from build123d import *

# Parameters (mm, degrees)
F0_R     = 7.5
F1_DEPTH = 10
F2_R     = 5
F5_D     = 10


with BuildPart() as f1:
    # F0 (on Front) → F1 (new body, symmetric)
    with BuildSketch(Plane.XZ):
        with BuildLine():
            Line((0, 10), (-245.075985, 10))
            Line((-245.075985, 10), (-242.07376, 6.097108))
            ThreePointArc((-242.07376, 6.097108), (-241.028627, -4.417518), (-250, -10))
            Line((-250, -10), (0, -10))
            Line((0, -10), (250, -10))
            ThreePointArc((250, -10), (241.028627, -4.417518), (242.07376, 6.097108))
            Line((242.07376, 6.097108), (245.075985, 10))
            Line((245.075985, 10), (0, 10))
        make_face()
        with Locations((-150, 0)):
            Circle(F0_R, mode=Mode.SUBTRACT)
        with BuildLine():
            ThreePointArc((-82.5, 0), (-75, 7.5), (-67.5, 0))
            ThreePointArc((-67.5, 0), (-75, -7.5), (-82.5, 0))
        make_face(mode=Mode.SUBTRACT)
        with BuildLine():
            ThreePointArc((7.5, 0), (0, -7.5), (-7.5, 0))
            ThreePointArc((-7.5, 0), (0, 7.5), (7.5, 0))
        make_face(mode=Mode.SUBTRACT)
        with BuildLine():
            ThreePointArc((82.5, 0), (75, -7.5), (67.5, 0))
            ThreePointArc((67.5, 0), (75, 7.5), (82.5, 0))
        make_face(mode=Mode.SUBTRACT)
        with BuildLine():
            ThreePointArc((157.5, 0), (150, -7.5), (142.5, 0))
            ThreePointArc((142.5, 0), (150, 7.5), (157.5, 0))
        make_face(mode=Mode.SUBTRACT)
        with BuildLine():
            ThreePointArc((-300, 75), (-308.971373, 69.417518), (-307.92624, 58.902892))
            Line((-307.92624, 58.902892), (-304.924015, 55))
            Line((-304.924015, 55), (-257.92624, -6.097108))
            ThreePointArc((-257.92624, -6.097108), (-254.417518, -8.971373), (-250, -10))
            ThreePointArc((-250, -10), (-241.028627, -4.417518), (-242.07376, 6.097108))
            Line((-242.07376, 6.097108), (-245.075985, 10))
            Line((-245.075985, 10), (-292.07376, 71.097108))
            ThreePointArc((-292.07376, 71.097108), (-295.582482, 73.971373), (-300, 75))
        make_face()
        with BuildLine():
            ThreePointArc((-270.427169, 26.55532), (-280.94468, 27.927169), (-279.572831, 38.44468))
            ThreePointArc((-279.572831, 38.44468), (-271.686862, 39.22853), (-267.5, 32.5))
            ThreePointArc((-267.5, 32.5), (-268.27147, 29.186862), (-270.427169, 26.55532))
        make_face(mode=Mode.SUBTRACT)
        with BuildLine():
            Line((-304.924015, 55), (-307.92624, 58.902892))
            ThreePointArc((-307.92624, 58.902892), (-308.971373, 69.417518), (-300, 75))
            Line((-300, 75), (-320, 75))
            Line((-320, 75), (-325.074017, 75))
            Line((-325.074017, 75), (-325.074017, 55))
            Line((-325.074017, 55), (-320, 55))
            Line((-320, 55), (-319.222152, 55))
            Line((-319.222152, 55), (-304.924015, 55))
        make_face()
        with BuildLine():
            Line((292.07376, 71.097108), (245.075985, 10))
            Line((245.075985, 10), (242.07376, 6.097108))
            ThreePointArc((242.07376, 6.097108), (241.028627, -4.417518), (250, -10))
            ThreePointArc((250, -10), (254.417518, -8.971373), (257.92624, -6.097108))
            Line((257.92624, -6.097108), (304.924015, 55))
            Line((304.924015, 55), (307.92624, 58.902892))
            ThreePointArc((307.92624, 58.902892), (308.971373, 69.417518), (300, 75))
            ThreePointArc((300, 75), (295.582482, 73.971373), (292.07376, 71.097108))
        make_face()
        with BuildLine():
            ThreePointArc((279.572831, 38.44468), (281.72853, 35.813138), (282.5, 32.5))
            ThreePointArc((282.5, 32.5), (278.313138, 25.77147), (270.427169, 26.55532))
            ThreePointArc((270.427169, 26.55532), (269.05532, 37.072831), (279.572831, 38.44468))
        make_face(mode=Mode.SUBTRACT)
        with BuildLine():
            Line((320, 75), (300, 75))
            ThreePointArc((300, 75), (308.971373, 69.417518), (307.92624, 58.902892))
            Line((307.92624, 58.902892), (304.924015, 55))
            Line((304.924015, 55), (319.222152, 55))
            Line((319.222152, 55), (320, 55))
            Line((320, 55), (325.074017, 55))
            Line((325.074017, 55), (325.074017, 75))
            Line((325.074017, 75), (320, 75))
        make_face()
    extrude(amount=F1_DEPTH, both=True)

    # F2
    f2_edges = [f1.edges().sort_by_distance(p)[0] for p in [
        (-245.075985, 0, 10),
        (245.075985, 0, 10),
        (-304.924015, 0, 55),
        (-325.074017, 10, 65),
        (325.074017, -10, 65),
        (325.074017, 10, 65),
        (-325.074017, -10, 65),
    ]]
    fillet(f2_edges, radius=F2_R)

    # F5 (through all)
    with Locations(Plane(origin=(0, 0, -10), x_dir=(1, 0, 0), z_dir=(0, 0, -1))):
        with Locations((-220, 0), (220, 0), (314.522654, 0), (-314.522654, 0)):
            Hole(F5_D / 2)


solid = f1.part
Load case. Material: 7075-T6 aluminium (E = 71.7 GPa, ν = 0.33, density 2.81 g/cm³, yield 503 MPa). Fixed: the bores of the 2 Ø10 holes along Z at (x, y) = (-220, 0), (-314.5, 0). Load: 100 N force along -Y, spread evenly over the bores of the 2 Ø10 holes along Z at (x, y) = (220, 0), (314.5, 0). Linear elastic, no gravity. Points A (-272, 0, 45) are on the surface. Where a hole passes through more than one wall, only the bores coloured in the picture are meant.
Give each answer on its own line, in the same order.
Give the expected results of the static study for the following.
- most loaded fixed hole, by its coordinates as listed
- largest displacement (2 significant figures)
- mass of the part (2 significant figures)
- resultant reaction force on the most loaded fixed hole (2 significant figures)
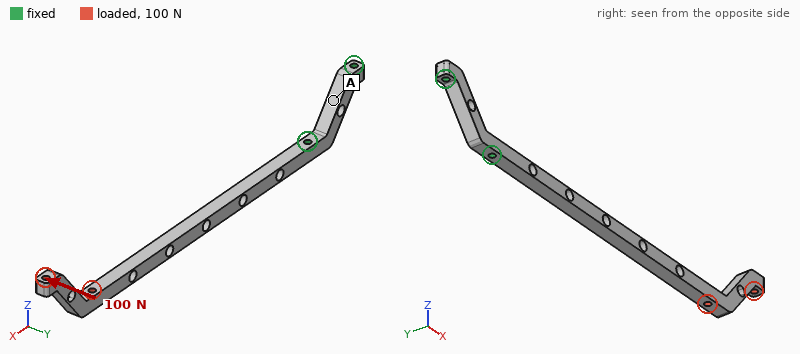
(-220, 0)
7.6 mm
710 g
130 N
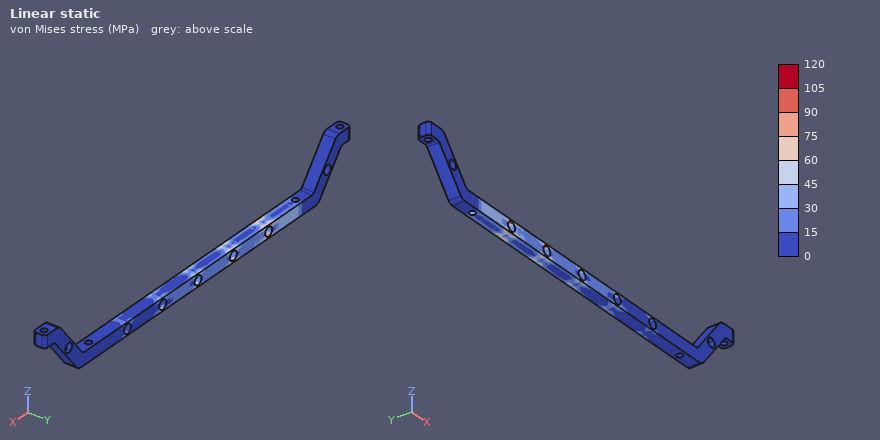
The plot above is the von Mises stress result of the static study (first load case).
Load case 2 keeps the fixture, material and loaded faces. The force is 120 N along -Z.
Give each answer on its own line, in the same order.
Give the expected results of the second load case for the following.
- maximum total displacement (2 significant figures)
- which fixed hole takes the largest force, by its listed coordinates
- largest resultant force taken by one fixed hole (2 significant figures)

6.4 mm
(-220, 0)
160 N
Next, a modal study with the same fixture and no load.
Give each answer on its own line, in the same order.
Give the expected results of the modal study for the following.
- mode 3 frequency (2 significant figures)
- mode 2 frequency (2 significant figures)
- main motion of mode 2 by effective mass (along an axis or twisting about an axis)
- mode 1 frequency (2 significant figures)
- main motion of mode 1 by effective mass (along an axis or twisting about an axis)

260 Hz
51 Hz
along Z
43 Hz
along Y
